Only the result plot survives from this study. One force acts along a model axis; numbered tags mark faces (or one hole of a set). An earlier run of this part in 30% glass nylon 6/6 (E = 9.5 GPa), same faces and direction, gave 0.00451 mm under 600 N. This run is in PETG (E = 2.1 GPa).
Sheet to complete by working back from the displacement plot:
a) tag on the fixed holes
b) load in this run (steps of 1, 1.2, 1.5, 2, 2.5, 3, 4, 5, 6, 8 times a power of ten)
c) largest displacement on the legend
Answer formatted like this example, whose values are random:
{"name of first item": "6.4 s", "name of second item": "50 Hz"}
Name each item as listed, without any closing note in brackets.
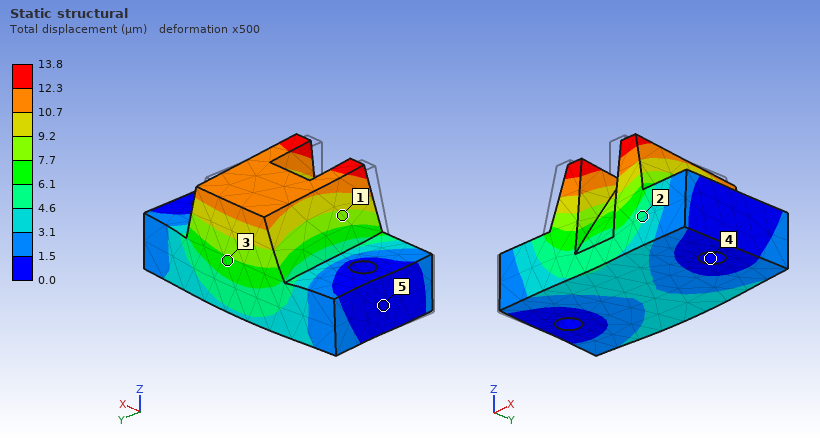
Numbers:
{"tag on the fixed holes": "4", "load in this run": "400 N", "largest displacement on the legend": "13.8 µm"}
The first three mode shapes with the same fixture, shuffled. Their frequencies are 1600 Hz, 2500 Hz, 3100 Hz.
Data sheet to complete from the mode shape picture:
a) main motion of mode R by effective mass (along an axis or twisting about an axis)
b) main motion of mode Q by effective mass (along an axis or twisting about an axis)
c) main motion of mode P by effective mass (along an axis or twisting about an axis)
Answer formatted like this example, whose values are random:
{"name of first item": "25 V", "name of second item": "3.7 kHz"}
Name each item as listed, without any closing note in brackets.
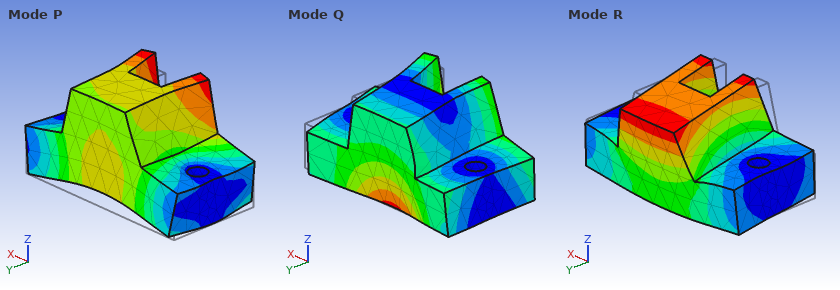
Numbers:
{"main motion of mode R by effective mass": "along Y", "main motion of mode Q by effective mass": "along Y", "main motion of mode P by effective mass": "along Z"}
